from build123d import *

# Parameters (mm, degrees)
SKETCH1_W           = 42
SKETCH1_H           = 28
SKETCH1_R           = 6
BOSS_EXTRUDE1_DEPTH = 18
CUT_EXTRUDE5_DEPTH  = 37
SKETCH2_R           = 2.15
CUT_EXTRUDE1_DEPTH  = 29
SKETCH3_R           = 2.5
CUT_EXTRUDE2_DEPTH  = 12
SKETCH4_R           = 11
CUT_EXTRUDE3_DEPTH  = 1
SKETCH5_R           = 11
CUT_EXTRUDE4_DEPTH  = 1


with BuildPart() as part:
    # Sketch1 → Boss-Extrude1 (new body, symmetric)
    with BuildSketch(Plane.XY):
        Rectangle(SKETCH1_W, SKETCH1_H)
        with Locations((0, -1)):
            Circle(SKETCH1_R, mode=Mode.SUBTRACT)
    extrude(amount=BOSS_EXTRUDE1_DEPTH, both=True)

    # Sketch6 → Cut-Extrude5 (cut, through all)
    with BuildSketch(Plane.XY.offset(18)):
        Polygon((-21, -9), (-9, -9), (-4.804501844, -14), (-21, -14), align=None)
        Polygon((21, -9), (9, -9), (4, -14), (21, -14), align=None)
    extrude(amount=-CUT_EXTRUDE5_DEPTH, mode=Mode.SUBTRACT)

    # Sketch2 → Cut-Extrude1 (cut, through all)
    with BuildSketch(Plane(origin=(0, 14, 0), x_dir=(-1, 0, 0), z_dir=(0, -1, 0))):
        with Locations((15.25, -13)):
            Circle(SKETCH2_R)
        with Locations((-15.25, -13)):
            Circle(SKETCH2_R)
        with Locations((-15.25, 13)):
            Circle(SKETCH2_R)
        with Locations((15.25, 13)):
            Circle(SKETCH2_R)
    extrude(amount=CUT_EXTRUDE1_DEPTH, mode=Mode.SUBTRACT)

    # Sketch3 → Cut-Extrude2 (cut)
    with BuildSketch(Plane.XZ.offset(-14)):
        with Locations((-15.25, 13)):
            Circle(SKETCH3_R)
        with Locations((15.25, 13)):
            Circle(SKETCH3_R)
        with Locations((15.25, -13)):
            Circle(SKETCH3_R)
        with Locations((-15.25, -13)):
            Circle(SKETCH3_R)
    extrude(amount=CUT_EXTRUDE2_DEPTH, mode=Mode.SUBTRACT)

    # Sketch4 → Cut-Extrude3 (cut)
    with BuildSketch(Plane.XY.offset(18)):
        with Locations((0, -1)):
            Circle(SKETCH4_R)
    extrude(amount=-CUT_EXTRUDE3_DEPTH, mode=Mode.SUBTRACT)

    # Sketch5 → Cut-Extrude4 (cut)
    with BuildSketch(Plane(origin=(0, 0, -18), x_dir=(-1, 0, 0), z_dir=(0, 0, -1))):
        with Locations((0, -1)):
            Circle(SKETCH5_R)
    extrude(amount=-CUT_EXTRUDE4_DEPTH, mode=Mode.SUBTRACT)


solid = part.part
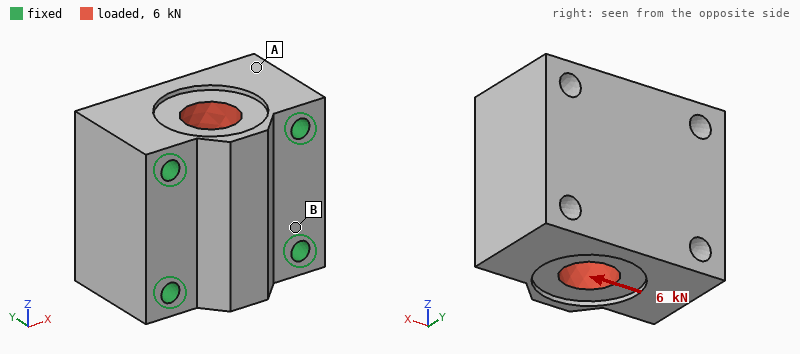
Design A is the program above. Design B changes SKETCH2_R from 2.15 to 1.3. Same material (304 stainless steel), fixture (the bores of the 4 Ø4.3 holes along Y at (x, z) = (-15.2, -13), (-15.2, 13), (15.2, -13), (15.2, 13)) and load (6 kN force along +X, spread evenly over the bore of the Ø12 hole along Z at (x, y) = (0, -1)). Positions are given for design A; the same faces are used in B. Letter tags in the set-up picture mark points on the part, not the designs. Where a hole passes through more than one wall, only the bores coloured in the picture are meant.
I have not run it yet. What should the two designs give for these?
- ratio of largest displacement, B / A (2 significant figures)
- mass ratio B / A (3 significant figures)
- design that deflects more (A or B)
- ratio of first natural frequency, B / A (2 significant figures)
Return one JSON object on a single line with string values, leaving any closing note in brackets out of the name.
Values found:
{"ratio of largest displacement, B / A": "1.2", "mass ratio B / A": "1.01", "design that deflects more": "B", "ratio of first natural frequency, B / A": "0.89"}
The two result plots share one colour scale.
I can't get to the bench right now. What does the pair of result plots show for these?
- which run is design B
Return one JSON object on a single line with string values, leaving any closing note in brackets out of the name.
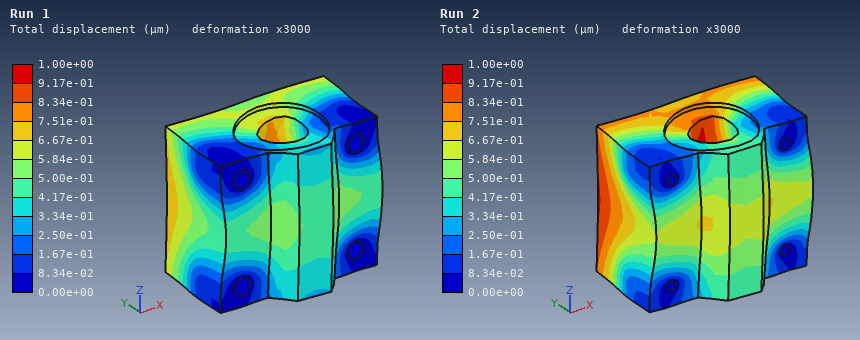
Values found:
{"which run is design B": "Run 2"}
